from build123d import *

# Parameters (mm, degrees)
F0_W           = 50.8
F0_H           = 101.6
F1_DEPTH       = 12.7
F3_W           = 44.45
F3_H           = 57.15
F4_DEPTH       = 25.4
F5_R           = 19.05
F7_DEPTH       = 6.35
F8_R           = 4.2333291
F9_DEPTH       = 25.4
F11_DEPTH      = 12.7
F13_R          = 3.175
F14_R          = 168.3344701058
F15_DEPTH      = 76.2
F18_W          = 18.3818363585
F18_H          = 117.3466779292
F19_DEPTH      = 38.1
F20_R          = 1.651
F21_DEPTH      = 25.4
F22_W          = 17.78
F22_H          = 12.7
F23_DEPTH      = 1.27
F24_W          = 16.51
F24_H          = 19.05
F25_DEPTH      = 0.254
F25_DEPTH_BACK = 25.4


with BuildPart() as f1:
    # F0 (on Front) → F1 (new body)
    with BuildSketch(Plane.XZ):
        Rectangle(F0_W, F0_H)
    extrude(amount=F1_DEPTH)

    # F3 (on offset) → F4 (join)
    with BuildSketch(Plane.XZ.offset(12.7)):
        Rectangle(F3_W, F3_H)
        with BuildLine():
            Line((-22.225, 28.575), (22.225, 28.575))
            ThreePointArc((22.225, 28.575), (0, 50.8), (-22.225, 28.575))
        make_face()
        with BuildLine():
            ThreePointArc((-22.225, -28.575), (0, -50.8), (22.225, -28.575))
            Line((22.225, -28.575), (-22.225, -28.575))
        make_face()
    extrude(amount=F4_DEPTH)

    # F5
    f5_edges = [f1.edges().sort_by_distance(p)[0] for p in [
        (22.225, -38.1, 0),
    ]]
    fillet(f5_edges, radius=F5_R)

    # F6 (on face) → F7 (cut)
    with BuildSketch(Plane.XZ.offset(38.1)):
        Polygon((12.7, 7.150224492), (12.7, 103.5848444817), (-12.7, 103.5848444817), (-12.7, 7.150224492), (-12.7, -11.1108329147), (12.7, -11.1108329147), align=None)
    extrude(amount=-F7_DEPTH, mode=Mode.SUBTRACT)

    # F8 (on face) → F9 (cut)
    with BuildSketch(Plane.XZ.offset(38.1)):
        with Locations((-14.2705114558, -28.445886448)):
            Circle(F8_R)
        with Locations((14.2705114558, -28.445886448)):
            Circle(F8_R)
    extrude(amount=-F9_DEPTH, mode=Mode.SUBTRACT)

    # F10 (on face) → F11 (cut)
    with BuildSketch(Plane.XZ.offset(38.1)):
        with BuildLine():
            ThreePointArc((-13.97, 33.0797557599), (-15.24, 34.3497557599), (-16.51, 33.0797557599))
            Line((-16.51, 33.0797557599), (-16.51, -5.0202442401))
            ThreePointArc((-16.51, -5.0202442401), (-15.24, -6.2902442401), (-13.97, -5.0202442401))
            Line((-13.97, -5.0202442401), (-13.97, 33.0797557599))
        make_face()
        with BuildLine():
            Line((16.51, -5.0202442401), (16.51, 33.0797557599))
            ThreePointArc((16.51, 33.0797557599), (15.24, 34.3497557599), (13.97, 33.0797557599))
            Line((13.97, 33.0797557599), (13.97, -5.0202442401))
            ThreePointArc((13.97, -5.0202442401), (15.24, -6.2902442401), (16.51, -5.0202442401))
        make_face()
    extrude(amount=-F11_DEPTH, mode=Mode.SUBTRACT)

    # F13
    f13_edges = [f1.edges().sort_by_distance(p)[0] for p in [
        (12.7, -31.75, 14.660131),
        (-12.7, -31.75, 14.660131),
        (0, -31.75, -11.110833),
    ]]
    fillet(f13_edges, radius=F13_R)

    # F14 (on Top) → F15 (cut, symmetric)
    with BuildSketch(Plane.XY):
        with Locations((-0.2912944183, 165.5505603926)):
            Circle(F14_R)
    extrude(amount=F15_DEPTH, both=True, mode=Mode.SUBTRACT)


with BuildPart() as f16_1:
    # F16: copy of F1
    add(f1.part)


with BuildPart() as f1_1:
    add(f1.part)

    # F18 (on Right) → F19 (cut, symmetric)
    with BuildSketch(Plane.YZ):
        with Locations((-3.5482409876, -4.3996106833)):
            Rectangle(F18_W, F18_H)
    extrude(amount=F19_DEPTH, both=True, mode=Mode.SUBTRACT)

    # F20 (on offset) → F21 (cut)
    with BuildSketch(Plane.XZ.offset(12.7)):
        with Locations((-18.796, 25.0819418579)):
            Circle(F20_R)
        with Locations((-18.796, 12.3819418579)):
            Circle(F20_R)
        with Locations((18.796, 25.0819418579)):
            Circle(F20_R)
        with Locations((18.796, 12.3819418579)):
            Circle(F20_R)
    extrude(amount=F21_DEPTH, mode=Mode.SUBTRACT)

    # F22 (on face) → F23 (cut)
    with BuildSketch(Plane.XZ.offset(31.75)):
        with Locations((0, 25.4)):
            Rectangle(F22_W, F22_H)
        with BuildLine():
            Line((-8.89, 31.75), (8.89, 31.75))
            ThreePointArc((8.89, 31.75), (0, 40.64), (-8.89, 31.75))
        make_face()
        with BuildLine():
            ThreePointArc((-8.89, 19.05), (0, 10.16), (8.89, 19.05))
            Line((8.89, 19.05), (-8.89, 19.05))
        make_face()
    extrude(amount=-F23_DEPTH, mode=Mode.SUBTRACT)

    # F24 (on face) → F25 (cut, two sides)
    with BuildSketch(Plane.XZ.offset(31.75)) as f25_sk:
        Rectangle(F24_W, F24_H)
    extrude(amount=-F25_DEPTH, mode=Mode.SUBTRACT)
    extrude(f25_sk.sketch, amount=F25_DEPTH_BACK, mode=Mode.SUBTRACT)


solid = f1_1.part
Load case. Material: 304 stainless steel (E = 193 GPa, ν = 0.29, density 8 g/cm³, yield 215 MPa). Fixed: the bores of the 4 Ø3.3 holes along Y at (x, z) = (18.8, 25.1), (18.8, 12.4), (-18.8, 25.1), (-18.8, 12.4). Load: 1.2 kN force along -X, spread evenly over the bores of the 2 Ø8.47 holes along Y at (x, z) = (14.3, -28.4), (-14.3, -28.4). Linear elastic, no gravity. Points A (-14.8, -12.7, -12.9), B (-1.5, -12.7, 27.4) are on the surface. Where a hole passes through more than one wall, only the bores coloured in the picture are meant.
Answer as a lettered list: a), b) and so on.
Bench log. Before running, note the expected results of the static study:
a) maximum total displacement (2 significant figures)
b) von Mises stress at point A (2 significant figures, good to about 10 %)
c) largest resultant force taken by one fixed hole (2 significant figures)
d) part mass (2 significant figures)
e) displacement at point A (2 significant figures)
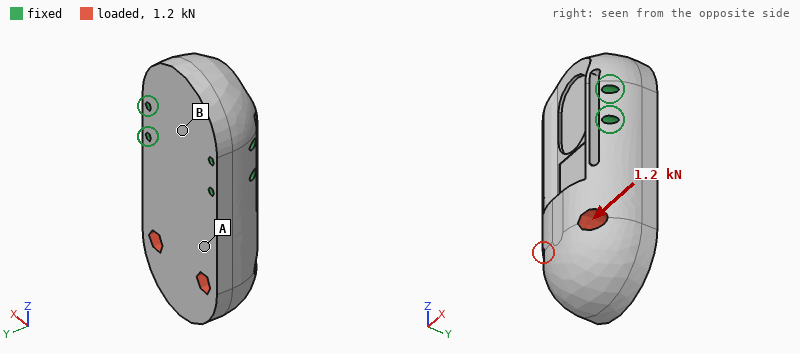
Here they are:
a) 3.4 µm
b) 3.2 MPa
c) 1.3 kN
d) 590 g
e) 1.3 µm
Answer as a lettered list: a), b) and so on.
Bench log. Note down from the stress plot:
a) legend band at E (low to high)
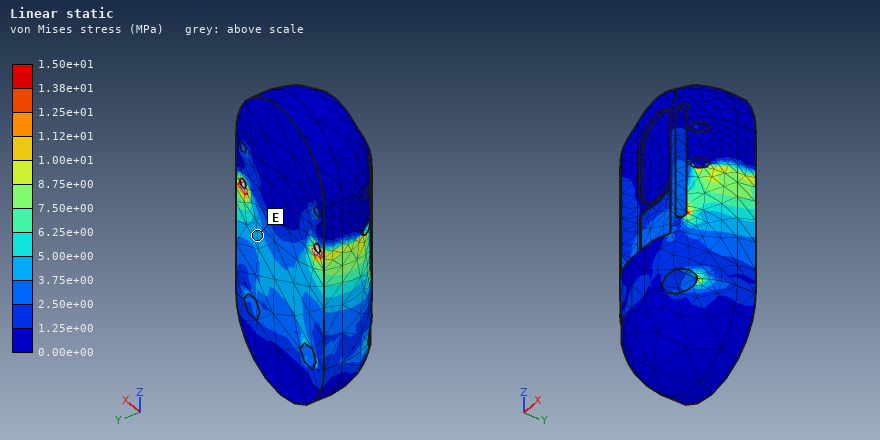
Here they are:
a) 3.75e+00 to 5.00e+00 MPa
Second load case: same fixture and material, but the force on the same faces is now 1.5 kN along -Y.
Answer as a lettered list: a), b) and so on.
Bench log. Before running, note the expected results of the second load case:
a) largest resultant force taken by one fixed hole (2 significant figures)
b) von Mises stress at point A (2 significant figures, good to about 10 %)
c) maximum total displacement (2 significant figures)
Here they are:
a) 1.4 kN
b) 8.5 MPa
c) 22 µm
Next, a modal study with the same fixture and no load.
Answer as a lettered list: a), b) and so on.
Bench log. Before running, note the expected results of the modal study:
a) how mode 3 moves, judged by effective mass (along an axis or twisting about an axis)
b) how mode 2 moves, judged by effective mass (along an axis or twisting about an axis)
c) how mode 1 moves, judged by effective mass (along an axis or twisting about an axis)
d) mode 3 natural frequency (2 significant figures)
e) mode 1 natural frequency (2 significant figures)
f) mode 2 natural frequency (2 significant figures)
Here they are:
a) twisting about Z
b) along X
c) along Y
d) 10 kHz
e) 3200 Hz
f) 7000 Hz
